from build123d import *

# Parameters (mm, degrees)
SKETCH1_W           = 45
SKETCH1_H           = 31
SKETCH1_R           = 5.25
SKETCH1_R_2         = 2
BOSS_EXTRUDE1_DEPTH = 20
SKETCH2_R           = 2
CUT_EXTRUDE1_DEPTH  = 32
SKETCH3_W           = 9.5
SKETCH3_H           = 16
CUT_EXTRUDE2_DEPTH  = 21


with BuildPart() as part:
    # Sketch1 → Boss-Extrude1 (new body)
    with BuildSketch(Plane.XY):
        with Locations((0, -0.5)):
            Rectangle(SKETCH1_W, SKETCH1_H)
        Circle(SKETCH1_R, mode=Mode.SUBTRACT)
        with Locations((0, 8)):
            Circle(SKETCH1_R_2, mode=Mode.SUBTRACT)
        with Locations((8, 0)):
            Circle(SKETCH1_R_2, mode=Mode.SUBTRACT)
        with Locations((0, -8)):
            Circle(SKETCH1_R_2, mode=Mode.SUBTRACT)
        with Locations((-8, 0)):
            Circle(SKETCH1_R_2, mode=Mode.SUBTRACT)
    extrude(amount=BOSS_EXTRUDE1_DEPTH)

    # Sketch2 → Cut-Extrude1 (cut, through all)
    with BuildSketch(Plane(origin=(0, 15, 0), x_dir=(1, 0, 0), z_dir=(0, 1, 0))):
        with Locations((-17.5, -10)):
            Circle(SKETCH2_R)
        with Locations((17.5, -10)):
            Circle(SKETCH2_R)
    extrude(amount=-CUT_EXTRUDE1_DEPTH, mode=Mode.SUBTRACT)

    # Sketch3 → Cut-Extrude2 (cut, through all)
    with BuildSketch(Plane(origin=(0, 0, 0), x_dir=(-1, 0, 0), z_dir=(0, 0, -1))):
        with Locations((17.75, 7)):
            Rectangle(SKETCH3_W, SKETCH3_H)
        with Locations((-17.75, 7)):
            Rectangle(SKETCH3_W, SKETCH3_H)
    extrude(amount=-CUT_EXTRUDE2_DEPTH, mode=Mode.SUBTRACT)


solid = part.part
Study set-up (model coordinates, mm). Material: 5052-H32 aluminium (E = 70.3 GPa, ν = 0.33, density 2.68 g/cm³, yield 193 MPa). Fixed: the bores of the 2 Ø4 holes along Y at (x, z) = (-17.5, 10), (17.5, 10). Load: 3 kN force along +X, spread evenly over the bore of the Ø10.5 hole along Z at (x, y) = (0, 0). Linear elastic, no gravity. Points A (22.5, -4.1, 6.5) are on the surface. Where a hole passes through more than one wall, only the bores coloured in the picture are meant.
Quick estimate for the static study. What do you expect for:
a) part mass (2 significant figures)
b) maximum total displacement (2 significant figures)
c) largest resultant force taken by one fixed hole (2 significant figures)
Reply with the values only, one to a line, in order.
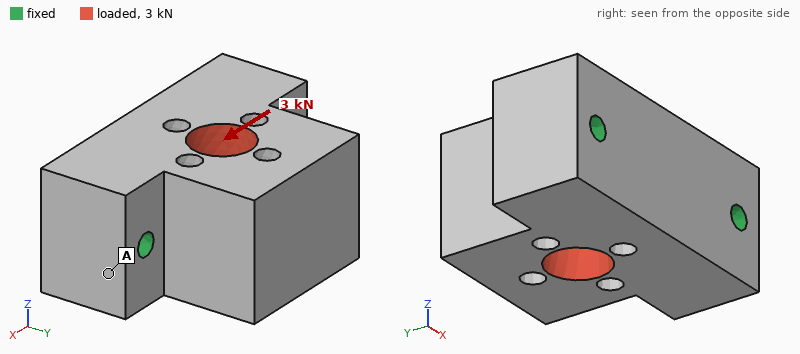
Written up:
50 g
6.0 µm
1.6 kN
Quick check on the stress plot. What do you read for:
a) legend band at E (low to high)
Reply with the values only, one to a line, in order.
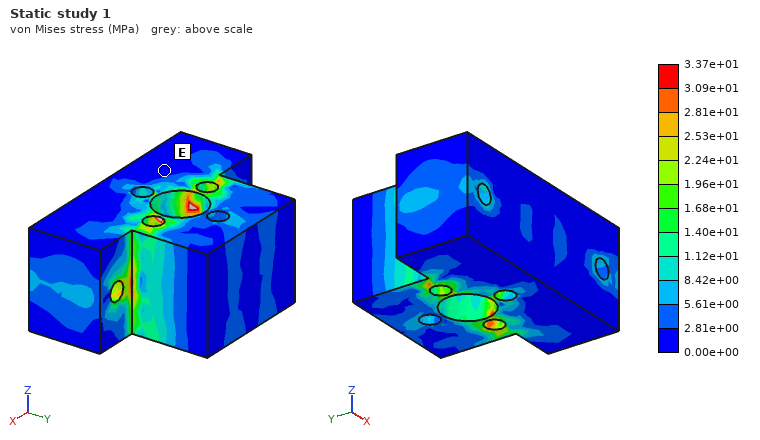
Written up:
0.00e+00 to 2.81e+00 MPa
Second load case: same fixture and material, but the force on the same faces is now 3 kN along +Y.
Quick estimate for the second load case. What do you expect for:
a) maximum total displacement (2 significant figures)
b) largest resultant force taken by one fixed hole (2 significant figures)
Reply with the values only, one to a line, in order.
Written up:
5.0 µm
1.5 kN
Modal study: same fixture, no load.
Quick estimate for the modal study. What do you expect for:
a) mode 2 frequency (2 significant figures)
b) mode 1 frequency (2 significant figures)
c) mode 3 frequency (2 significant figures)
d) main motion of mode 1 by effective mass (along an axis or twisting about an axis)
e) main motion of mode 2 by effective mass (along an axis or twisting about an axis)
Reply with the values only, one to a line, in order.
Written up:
19 kHz
12 kHz
24 kHz
along Z
along X
